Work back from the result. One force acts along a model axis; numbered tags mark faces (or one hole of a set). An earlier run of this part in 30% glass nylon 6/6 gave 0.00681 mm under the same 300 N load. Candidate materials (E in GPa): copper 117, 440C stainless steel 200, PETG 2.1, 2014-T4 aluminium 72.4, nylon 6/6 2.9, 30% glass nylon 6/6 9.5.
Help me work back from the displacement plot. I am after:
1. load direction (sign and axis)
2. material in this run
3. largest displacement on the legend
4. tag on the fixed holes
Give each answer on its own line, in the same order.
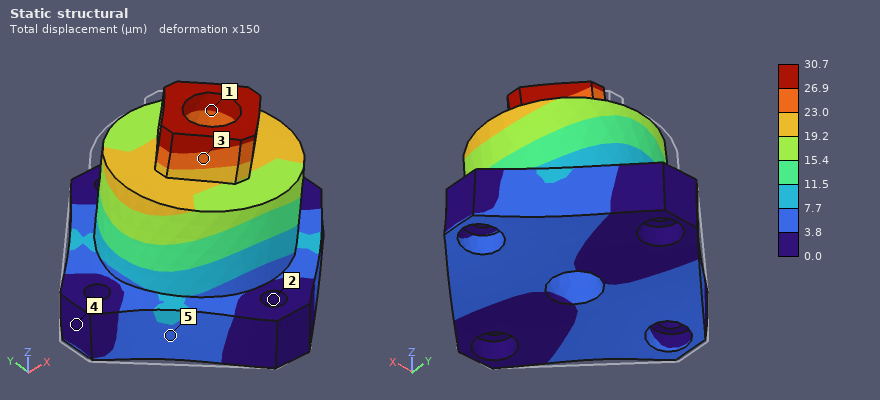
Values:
+X
PETG
30.7 µm
2
